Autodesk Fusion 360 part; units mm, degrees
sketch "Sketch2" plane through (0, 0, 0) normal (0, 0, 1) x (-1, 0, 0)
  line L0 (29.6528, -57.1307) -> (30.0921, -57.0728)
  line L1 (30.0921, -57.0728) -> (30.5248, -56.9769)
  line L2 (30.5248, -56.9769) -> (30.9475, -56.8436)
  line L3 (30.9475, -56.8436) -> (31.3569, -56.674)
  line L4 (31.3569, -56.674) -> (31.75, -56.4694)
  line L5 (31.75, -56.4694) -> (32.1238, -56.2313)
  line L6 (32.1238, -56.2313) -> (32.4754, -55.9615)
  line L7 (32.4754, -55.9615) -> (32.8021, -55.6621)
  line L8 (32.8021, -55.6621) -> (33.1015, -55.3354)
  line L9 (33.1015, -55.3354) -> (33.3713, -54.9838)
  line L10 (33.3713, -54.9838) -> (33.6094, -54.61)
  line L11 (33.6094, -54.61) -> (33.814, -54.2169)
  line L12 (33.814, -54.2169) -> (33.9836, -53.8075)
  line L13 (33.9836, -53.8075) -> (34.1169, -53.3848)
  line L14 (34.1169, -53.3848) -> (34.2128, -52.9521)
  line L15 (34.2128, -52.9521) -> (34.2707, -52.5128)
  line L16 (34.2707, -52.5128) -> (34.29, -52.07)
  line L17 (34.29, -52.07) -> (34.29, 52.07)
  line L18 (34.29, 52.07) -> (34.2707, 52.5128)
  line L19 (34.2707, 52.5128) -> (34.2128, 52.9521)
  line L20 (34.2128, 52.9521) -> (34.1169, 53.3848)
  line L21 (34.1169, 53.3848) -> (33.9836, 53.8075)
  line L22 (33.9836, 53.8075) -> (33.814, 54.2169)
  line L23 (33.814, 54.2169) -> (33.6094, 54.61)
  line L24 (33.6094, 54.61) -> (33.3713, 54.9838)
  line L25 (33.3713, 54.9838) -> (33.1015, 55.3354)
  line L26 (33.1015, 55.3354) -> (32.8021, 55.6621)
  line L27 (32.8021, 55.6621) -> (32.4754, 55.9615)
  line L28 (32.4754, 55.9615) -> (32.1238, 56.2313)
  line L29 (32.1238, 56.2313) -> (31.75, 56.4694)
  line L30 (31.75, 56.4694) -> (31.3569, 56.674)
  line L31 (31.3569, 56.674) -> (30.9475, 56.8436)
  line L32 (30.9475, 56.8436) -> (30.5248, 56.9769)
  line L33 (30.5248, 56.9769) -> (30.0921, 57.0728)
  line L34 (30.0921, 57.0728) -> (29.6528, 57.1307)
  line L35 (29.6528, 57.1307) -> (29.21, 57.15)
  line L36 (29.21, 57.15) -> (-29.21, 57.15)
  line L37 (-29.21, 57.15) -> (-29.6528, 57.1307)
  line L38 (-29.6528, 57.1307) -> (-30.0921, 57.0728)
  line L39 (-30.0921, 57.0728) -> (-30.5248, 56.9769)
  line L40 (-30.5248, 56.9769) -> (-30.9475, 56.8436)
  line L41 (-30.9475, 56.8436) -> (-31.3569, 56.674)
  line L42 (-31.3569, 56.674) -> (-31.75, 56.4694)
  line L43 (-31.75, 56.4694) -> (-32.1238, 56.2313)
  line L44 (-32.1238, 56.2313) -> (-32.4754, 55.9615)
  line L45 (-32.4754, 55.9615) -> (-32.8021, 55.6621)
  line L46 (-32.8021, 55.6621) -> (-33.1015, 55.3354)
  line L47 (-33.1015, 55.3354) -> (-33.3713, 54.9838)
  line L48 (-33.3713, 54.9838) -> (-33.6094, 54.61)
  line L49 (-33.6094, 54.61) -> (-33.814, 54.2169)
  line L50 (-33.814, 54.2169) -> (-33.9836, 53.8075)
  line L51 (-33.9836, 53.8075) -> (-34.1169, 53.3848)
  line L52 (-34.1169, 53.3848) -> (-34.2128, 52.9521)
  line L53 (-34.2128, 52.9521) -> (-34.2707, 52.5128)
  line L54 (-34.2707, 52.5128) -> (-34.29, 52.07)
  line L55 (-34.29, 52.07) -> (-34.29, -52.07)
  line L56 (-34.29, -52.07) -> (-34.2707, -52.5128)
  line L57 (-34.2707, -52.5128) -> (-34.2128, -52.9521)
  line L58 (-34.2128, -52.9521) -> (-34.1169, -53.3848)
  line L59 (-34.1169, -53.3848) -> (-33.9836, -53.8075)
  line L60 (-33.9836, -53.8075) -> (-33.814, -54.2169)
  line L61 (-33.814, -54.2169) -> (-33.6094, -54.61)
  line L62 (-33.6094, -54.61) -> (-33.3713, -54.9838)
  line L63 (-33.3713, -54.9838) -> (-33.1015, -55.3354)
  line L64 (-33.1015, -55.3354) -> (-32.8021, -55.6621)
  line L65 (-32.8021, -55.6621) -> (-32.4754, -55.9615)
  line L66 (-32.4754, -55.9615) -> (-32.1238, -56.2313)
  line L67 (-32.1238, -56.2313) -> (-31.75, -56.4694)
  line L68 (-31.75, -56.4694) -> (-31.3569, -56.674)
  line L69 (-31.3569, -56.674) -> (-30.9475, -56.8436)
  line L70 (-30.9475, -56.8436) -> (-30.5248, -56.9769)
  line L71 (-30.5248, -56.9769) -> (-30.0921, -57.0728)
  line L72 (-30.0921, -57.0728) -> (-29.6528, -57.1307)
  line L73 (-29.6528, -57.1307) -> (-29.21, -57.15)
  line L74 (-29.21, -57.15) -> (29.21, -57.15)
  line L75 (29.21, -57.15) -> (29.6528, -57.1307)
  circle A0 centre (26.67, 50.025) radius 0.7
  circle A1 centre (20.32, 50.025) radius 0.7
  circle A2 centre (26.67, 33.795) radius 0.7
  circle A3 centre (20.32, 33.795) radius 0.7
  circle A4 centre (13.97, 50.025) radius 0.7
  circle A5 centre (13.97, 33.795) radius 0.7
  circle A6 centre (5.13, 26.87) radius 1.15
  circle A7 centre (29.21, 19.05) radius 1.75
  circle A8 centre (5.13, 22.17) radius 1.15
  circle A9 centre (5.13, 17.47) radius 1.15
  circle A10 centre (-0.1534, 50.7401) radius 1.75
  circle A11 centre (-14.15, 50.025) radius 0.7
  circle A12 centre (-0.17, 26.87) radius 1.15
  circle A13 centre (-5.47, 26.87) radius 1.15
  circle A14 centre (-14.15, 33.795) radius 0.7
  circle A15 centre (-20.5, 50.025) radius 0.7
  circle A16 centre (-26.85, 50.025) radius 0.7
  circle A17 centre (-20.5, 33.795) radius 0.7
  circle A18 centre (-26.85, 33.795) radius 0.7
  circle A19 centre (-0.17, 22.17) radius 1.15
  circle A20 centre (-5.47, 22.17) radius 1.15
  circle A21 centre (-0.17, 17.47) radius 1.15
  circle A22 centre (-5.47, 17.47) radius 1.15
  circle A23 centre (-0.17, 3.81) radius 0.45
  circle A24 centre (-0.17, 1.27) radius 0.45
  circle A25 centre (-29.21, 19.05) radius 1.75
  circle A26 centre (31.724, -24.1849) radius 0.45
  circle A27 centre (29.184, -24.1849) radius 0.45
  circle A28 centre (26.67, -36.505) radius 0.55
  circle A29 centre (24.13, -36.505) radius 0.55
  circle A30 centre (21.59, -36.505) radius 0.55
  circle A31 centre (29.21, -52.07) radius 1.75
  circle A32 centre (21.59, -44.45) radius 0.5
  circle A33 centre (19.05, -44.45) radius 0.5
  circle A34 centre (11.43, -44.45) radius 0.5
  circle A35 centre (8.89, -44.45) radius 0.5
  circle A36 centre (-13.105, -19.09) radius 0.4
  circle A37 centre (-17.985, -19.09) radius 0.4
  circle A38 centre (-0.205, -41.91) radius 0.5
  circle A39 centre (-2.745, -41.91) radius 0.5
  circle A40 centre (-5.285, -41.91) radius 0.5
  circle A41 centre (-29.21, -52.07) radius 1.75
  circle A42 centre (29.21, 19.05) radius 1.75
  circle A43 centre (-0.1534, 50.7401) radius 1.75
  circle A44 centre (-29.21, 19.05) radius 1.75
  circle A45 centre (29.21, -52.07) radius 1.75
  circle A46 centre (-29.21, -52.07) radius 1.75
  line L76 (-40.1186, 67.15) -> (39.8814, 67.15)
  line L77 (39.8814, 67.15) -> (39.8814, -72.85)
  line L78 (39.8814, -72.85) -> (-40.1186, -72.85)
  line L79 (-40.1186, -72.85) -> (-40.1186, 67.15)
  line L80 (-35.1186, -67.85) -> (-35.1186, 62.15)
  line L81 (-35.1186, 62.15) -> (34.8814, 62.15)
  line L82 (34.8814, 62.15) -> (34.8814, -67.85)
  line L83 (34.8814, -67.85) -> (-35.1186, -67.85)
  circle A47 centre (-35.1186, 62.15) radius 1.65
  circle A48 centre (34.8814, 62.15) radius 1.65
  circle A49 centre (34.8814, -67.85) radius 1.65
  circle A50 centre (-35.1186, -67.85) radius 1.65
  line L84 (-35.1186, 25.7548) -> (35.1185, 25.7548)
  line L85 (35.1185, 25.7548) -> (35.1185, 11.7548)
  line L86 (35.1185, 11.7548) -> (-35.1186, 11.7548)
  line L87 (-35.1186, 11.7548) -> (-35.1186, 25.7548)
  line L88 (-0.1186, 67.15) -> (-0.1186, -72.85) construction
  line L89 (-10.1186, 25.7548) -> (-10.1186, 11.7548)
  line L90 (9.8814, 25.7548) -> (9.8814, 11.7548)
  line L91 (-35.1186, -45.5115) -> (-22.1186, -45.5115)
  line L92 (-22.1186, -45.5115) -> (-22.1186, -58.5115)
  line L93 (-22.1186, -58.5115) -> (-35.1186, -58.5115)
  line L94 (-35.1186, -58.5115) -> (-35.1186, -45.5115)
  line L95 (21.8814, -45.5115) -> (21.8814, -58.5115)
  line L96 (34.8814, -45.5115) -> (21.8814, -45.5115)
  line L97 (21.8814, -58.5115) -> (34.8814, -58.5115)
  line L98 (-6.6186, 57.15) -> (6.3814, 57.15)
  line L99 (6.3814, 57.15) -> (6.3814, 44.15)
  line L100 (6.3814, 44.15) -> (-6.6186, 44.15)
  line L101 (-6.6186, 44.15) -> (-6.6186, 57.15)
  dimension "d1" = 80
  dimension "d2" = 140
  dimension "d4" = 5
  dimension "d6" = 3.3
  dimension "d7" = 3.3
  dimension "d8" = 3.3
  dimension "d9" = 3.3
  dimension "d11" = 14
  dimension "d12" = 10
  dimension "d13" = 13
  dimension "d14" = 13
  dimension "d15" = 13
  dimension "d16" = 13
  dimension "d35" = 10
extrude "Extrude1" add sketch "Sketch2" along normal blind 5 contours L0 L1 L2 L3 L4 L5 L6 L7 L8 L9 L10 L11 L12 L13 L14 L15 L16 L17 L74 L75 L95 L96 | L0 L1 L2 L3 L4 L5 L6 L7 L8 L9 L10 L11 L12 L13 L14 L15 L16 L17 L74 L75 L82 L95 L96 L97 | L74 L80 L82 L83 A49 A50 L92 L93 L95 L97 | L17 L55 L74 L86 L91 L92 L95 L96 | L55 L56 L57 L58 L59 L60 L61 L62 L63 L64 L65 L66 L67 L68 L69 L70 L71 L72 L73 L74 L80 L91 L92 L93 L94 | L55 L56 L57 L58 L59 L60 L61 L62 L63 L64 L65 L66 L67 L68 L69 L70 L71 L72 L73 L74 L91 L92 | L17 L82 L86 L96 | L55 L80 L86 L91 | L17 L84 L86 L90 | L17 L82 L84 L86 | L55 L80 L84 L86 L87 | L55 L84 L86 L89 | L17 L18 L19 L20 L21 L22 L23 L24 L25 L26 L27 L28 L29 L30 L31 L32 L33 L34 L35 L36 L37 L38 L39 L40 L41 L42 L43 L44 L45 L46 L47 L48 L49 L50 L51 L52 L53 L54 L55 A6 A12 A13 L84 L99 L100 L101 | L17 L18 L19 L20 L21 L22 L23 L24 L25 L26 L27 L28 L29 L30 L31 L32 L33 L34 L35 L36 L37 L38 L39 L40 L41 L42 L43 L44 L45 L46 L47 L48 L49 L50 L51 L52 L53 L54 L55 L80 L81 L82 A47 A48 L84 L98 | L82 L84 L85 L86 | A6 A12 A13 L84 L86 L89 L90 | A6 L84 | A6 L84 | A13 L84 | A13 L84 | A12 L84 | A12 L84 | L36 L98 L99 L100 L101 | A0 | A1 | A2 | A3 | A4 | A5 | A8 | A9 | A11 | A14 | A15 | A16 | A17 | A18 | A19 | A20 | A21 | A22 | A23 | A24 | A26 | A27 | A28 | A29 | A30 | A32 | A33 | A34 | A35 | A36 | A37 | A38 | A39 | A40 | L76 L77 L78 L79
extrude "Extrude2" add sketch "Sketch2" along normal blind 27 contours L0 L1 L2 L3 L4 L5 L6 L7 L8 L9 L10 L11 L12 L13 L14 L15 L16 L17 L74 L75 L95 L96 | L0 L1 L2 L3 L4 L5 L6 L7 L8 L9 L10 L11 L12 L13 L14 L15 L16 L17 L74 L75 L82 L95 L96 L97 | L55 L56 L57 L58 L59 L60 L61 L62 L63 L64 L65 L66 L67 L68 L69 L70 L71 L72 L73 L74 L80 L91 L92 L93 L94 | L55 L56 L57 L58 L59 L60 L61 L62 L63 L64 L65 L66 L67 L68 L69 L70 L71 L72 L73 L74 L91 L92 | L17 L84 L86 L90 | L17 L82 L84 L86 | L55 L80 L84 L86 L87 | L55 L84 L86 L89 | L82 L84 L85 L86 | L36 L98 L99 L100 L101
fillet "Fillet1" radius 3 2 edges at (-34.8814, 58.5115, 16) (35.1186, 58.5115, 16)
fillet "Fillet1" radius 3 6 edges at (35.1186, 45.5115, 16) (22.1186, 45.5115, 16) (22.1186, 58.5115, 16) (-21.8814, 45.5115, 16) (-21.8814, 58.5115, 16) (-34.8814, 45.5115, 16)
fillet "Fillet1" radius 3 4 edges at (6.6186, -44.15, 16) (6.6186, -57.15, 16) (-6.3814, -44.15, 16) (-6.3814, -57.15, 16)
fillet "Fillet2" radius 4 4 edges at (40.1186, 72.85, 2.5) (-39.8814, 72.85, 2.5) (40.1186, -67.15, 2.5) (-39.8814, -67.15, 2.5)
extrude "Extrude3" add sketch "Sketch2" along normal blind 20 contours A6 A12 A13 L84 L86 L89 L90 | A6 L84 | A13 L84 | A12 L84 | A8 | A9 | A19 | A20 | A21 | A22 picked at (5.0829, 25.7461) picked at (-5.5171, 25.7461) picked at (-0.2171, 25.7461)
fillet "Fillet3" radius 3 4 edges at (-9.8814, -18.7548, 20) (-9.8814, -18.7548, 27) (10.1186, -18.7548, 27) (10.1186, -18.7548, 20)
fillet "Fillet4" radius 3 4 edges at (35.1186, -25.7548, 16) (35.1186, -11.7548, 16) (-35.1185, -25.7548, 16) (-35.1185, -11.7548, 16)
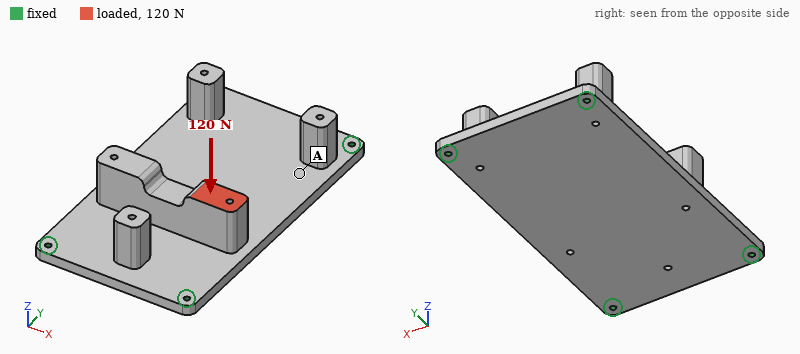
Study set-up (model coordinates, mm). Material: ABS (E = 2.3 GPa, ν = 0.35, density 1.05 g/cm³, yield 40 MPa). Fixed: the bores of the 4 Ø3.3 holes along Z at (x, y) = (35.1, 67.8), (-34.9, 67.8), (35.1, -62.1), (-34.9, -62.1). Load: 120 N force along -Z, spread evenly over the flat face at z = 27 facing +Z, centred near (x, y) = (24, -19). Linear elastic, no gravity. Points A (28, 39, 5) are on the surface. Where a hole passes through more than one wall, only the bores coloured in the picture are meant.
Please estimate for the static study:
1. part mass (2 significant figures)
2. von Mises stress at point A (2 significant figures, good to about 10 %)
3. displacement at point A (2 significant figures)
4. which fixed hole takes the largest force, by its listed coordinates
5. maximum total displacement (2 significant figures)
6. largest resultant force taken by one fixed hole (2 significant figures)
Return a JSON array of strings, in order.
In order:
["89 g", "1.8 MPa", "0.42 mm", "(35.1, -62.1)", "1.1 mm", "77 N"]
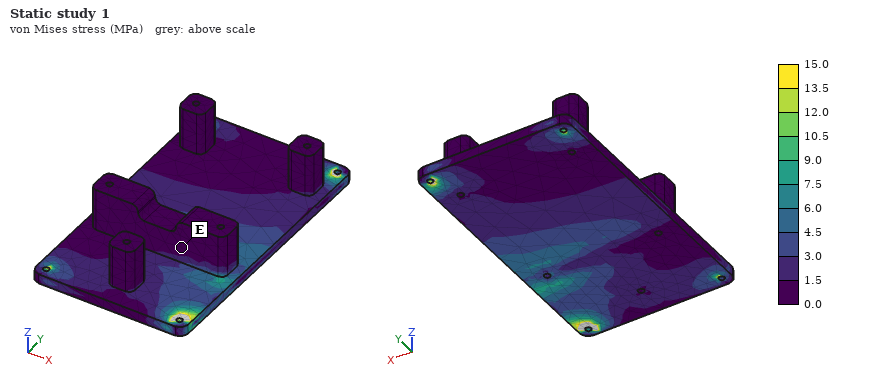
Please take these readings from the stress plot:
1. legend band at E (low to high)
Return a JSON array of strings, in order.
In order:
["0.0 to 1.5 MPa"]
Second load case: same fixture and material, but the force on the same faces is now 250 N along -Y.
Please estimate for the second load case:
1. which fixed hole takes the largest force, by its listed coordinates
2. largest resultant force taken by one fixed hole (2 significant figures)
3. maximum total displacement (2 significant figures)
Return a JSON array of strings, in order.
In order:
["(35.1, -62.1)", "100 N", "1.1 mm"]
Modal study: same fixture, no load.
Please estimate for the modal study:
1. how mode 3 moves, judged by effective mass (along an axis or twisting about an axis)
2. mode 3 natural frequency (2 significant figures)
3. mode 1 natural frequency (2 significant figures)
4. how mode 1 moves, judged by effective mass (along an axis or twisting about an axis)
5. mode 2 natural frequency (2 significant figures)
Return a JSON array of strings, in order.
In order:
["twisting about X", "780 Hz", "290 Hz", "along Z", "540 Hz"]
